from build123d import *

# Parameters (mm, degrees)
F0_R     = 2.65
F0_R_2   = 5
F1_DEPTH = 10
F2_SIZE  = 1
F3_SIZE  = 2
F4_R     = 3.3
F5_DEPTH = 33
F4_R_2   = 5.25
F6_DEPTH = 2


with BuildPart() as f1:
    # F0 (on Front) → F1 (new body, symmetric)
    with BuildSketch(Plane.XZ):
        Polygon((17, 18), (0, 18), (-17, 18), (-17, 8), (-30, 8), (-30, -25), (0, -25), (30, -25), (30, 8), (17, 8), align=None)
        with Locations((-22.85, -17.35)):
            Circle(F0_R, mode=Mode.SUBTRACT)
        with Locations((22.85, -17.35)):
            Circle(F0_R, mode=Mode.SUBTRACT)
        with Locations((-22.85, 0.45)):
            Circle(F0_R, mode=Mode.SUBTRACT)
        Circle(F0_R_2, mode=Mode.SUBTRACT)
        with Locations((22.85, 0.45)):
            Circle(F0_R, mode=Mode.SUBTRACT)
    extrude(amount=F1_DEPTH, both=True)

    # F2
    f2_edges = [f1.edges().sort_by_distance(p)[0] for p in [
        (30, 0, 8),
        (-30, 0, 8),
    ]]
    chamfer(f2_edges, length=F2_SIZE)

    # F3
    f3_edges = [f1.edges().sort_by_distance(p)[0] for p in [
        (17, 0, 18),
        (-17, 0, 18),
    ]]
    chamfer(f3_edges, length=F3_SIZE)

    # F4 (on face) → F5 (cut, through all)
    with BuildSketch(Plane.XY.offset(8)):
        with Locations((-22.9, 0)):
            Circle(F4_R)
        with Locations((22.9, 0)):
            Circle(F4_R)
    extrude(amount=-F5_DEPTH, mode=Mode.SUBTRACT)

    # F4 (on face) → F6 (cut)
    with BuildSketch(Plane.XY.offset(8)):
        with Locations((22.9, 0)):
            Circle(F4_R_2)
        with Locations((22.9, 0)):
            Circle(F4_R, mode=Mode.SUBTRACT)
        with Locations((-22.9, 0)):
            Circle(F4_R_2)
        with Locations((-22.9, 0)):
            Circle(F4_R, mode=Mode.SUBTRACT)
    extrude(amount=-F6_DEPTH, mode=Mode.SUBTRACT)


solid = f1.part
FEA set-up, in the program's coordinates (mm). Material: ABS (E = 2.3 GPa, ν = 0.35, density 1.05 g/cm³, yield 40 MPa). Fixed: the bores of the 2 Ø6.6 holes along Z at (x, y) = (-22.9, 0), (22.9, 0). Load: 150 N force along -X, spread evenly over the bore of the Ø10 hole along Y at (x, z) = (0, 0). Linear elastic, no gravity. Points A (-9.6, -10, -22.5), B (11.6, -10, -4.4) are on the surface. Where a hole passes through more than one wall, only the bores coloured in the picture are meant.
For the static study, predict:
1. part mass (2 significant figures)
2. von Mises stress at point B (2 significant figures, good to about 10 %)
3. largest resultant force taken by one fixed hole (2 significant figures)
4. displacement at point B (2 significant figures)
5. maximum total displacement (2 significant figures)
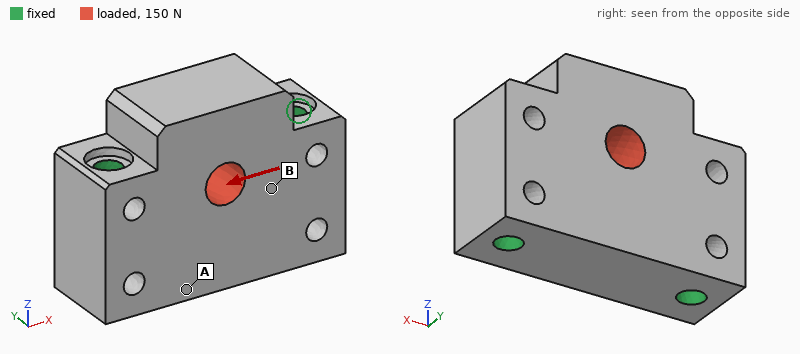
43 g
0.17 MPa
77 N
0.95 µm
2.3 µm
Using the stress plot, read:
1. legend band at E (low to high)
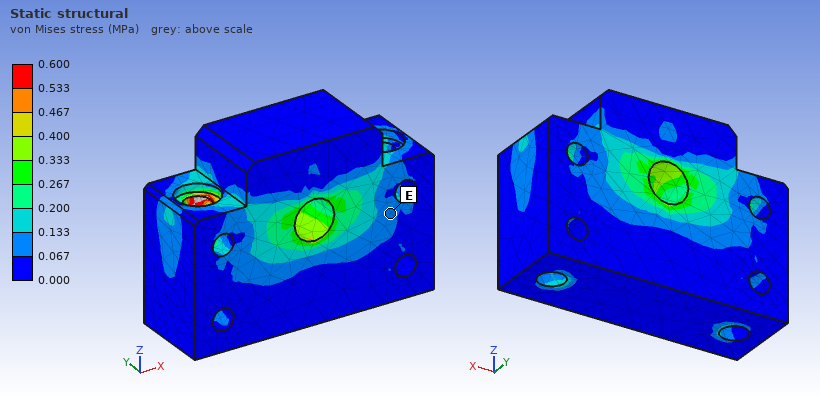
0.067 to 0.133 MPa
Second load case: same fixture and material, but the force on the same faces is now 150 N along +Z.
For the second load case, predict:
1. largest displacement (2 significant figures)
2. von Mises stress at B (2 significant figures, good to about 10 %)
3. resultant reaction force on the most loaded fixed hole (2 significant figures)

3.8 µm
0.18 MPa
77 N
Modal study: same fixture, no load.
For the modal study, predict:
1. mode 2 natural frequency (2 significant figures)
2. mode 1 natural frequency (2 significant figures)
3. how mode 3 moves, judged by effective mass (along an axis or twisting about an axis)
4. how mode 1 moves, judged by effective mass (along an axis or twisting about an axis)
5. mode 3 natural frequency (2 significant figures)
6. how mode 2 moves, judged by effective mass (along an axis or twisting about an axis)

7300 Hz
4700 Hz
along Z
along Y
8200 Hz
along Y
